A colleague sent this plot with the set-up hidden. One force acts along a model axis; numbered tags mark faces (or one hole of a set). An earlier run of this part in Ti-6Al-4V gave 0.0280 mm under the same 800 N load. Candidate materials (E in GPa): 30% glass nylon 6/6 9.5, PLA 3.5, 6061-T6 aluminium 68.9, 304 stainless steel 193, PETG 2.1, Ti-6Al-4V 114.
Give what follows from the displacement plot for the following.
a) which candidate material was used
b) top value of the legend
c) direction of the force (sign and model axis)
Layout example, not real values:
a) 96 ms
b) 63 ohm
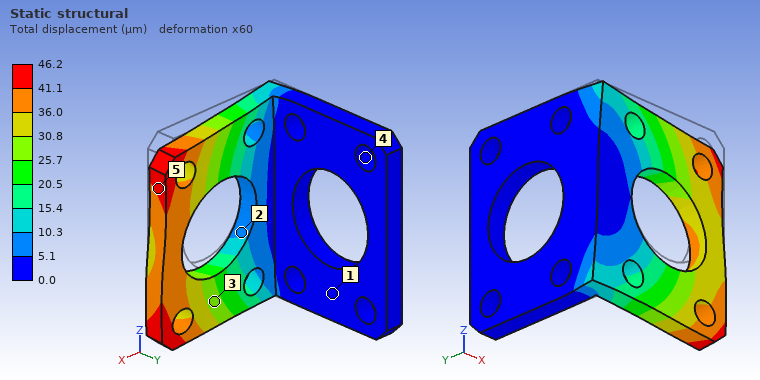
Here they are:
a) 6061-T6 aluminium
b) 46.2 µm
c) -Z
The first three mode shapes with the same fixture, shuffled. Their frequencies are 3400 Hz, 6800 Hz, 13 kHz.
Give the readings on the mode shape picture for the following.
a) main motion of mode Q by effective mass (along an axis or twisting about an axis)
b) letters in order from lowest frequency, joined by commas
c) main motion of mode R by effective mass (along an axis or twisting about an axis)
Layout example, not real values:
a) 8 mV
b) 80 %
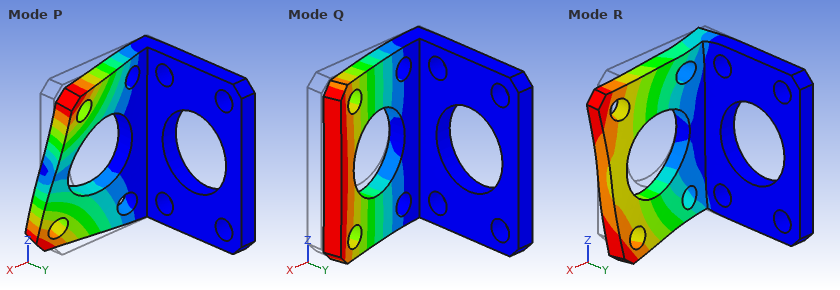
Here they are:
a) along Y
b) Q, P, R
c) along Z
